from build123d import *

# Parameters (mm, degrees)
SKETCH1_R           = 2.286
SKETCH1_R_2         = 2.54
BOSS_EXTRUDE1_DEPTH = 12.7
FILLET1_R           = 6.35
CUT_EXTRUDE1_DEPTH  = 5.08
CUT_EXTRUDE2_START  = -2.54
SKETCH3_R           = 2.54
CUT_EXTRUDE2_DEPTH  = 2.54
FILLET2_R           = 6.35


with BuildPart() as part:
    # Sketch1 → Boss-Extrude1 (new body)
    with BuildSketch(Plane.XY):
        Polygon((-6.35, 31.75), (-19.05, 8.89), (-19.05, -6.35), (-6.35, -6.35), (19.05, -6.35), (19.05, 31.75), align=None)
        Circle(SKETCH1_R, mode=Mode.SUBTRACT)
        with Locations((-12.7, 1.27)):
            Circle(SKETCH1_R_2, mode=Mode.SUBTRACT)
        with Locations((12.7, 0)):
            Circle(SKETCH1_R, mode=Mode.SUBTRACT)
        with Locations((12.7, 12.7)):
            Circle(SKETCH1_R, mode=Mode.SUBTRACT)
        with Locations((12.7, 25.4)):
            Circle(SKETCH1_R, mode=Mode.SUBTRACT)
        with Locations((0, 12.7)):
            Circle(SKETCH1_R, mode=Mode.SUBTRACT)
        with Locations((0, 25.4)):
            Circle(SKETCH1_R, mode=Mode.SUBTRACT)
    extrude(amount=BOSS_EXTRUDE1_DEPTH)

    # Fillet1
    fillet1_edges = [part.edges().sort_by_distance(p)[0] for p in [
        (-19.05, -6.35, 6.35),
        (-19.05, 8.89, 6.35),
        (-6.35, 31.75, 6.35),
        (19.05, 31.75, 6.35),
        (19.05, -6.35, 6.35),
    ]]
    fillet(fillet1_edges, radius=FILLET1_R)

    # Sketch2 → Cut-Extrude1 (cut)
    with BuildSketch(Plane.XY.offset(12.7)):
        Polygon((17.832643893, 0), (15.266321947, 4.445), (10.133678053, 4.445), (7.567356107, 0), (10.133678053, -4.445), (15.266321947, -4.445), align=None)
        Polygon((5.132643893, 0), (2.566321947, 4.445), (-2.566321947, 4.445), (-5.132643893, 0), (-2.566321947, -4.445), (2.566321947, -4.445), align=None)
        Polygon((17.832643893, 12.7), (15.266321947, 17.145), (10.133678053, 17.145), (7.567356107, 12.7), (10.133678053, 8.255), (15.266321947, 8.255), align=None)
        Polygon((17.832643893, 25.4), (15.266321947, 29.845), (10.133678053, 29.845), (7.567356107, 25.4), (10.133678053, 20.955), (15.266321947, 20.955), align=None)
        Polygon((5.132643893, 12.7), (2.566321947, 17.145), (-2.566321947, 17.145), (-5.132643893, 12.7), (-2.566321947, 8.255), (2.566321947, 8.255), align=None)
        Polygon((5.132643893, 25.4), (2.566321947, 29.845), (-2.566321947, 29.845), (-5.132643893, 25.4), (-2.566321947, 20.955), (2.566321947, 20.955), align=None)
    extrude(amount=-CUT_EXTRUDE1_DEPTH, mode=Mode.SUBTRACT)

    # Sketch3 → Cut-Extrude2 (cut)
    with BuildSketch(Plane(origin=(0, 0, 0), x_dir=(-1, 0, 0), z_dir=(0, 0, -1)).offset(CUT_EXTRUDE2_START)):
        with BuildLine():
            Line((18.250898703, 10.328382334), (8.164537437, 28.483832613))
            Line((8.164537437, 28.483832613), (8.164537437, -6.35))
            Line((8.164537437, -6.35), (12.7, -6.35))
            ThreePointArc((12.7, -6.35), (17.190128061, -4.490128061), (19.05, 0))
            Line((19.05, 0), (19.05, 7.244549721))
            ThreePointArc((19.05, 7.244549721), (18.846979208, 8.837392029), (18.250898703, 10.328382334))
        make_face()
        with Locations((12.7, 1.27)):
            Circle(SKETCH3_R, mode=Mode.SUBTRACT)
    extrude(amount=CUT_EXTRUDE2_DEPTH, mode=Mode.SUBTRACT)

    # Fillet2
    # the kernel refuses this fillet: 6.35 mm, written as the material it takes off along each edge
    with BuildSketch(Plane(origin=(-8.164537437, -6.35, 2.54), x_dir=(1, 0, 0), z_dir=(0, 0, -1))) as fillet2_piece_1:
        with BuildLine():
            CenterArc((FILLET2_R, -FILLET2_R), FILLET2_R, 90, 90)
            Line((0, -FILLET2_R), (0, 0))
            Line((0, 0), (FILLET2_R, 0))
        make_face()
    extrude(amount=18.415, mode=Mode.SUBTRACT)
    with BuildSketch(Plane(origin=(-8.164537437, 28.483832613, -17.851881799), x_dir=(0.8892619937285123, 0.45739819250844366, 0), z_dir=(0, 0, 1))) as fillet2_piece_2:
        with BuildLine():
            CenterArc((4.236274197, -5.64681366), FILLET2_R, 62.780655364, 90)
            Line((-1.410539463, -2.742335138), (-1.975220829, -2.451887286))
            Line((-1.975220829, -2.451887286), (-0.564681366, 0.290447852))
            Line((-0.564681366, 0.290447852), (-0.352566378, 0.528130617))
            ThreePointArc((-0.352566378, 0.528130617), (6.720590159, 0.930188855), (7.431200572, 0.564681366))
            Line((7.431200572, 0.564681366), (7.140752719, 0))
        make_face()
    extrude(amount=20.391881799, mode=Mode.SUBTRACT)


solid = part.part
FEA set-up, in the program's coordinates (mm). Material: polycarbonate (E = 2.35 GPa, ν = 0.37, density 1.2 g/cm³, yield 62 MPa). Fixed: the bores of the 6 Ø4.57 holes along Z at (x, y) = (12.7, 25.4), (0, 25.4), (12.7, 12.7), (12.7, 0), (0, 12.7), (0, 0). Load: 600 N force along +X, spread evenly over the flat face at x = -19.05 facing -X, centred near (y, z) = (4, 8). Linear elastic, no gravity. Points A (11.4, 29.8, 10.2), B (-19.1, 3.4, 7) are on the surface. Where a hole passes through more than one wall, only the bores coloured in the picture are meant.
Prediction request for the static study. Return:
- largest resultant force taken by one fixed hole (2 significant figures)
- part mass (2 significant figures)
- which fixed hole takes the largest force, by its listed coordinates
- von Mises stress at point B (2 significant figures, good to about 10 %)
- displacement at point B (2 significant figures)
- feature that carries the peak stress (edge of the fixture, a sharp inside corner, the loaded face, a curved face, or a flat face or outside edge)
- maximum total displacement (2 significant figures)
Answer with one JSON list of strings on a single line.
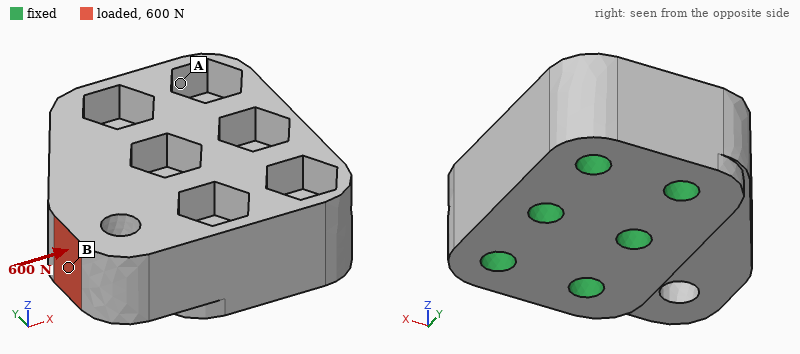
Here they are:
["320 N", "15 g", "(0, 0)", "7.1 MPa", "78 µm", "a curved face", "100 µm"]
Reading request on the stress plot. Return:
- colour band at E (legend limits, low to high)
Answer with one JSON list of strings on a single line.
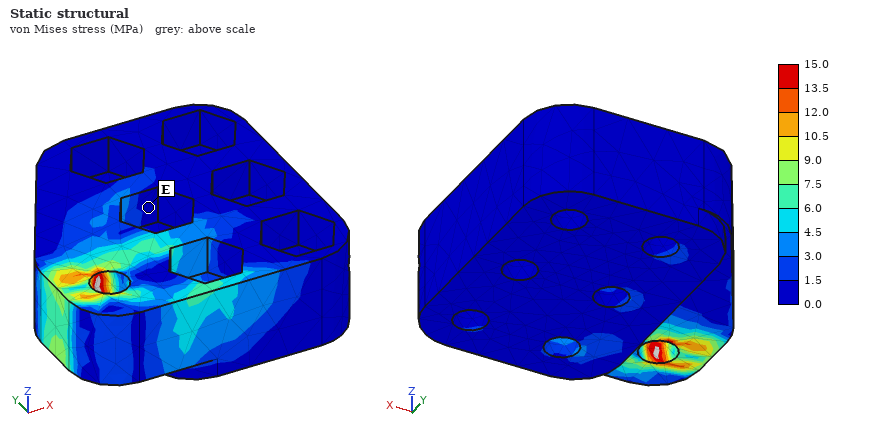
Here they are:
["0.0 to 1.5 MPa"]
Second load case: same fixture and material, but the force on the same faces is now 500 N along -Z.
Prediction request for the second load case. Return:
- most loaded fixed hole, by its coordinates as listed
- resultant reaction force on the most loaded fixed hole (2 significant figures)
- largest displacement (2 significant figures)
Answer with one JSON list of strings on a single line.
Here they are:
["(0, 0)", "420 N", "0.42 mm"]
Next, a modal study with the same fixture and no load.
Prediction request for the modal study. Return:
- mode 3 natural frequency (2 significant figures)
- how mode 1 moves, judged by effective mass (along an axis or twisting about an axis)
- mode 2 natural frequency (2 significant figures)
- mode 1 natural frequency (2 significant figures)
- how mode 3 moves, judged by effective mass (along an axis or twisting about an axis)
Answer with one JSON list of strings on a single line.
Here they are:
["10 kHz", "along Z", "9900 Hz", "5700 Hz", "along Y"]
